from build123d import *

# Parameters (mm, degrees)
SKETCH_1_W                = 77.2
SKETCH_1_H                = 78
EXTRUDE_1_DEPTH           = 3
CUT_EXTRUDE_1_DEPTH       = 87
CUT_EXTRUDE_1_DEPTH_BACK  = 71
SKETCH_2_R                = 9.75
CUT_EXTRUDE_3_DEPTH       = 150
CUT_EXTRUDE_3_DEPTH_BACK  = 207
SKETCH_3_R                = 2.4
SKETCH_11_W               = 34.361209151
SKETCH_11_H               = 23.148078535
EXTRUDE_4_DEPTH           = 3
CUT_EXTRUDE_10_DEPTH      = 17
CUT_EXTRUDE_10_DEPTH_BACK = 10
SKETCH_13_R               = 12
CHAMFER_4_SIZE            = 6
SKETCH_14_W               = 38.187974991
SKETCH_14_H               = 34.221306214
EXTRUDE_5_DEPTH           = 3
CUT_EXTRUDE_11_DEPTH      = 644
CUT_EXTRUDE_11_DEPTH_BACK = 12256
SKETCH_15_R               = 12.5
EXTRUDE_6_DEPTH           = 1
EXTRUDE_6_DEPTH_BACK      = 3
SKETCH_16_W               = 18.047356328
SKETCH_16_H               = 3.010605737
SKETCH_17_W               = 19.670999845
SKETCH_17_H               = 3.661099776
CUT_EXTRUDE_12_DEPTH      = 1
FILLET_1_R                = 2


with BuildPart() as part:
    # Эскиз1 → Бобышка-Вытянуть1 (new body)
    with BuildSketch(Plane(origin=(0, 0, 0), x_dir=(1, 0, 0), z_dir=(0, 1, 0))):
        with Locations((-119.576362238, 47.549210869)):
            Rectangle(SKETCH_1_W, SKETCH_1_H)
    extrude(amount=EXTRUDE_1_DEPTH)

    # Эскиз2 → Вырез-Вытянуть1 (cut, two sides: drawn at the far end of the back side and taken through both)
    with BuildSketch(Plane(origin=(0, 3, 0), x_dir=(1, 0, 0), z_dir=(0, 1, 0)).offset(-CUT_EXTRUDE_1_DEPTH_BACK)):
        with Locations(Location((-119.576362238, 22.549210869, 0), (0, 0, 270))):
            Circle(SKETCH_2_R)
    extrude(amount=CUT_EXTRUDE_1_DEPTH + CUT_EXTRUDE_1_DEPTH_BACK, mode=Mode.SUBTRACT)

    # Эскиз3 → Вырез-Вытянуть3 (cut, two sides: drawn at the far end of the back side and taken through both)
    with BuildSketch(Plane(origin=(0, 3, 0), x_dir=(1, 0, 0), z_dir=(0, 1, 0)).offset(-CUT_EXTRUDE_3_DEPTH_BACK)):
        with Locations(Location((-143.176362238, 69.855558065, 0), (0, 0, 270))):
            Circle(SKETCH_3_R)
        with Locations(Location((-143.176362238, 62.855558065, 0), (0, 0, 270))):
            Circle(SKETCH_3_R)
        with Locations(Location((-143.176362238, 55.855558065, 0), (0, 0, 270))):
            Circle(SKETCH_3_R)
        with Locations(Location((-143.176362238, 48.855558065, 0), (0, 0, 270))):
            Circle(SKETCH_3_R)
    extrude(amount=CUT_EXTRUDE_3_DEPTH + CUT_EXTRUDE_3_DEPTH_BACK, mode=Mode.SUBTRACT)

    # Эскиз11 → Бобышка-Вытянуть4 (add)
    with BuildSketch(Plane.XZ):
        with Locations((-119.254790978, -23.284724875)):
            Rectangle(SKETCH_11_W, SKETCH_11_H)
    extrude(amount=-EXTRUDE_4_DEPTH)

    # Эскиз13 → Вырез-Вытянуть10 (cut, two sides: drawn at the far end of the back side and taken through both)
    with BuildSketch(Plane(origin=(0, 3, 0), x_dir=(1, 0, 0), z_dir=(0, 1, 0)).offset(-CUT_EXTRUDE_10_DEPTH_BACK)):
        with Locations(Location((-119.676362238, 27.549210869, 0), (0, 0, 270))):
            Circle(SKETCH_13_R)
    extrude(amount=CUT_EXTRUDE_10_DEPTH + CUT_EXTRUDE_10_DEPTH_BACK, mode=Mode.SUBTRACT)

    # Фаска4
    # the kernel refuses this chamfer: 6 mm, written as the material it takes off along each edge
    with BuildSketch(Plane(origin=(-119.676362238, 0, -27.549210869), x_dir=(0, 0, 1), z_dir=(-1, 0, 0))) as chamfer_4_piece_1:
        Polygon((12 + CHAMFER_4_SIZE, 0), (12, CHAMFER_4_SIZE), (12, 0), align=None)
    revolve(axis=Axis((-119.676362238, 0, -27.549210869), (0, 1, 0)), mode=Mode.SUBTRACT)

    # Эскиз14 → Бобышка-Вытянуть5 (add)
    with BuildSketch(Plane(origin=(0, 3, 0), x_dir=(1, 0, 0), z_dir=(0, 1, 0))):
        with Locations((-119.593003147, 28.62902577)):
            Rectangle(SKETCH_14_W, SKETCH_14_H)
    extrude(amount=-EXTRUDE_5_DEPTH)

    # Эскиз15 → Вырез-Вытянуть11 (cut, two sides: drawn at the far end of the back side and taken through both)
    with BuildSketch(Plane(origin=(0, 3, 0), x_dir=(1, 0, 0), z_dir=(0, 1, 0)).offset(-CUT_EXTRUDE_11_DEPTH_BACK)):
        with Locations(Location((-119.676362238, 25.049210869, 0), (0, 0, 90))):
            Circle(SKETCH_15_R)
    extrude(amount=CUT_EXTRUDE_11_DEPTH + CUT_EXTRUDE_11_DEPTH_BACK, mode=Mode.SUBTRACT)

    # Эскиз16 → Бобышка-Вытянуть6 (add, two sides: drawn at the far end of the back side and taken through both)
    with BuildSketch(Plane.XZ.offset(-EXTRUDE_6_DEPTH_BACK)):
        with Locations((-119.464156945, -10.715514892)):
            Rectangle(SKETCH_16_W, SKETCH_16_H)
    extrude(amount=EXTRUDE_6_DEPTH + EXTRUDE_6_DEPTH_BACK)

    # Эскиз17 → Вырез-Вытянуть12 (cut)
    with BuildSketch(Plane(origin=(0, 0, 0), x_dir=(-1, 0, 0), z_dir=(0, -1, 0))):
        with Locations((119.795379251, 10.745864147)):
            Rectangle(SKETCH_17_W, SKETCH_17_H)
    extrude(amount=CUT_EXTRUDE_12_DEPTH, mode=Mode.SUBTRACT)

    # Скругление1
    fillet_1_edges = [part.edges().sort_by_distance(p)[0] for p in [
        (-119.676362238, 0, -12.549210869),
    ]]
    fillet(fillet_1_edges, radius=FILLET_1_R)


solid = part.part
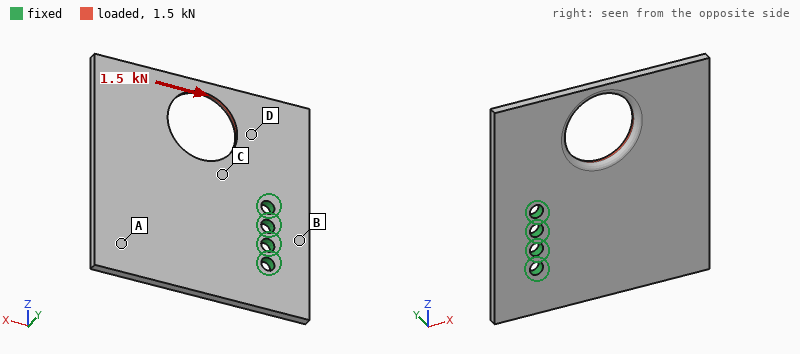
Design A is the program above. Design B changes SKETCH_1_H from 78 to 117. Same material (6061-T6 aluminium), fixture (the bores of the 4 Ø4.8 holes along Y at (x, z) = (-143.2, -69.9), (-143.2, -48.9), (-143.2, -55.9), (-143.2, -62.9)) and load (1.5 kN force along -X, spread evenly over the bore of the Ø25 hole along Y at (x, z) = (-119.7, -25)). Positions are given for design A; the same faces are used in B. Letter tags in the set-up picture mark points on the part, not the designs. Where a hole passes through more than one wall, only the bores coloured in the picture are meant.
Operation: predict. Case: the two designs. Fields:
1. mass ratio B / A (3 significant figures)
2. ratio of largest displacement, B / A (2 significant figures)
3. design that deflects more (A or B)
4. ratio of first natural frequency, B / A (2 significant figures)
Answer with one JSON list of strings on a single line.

["1.55", "0.88", "A", "0.78"]
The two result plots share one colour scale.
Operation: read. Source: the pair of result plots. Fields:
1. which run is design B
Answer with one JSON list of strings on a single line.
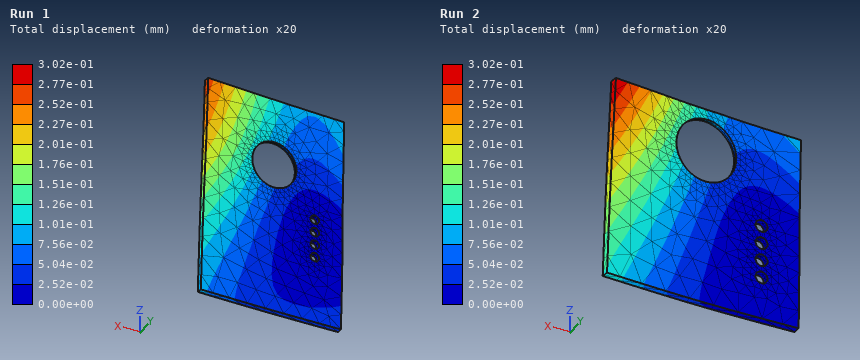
["Run 1"]
